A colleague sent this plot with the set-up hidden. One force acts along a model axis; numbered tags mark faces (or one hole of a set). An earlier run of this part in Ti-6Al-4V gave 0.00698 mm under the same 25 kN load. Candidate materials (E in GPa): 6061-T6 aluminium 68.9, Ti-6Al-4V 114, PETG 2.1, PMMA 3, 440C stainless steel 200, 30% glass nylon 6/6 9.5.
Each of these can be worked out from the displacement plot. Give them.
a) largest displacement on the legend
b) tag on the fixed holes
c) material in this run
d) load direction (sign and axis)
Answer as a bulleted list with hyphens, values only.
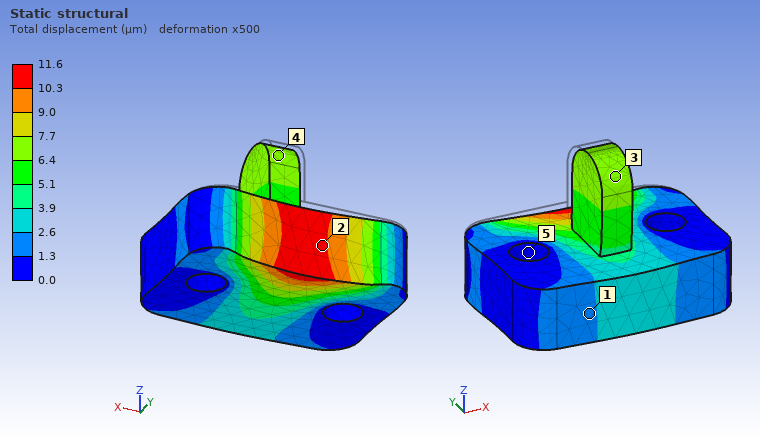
- 11.6 µm
- 5
- 6061-T6 aluminium
- -Y
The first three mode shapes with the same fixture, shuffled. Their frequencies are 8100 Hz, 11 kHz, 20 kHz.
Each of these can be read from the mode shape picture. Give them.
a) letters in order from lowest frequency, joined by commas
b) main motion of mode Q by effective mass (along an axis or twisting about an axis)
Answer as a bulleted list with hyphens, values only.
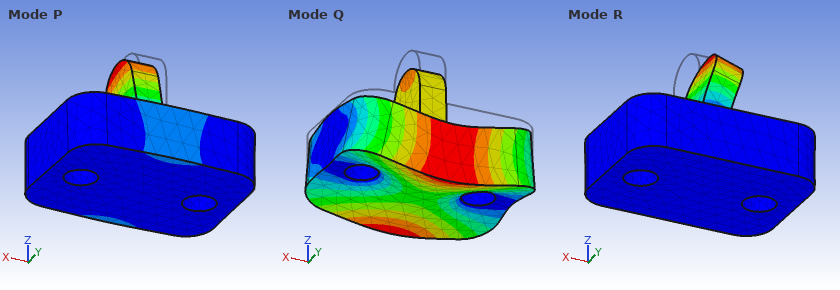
- R, P, Q
- along Z
